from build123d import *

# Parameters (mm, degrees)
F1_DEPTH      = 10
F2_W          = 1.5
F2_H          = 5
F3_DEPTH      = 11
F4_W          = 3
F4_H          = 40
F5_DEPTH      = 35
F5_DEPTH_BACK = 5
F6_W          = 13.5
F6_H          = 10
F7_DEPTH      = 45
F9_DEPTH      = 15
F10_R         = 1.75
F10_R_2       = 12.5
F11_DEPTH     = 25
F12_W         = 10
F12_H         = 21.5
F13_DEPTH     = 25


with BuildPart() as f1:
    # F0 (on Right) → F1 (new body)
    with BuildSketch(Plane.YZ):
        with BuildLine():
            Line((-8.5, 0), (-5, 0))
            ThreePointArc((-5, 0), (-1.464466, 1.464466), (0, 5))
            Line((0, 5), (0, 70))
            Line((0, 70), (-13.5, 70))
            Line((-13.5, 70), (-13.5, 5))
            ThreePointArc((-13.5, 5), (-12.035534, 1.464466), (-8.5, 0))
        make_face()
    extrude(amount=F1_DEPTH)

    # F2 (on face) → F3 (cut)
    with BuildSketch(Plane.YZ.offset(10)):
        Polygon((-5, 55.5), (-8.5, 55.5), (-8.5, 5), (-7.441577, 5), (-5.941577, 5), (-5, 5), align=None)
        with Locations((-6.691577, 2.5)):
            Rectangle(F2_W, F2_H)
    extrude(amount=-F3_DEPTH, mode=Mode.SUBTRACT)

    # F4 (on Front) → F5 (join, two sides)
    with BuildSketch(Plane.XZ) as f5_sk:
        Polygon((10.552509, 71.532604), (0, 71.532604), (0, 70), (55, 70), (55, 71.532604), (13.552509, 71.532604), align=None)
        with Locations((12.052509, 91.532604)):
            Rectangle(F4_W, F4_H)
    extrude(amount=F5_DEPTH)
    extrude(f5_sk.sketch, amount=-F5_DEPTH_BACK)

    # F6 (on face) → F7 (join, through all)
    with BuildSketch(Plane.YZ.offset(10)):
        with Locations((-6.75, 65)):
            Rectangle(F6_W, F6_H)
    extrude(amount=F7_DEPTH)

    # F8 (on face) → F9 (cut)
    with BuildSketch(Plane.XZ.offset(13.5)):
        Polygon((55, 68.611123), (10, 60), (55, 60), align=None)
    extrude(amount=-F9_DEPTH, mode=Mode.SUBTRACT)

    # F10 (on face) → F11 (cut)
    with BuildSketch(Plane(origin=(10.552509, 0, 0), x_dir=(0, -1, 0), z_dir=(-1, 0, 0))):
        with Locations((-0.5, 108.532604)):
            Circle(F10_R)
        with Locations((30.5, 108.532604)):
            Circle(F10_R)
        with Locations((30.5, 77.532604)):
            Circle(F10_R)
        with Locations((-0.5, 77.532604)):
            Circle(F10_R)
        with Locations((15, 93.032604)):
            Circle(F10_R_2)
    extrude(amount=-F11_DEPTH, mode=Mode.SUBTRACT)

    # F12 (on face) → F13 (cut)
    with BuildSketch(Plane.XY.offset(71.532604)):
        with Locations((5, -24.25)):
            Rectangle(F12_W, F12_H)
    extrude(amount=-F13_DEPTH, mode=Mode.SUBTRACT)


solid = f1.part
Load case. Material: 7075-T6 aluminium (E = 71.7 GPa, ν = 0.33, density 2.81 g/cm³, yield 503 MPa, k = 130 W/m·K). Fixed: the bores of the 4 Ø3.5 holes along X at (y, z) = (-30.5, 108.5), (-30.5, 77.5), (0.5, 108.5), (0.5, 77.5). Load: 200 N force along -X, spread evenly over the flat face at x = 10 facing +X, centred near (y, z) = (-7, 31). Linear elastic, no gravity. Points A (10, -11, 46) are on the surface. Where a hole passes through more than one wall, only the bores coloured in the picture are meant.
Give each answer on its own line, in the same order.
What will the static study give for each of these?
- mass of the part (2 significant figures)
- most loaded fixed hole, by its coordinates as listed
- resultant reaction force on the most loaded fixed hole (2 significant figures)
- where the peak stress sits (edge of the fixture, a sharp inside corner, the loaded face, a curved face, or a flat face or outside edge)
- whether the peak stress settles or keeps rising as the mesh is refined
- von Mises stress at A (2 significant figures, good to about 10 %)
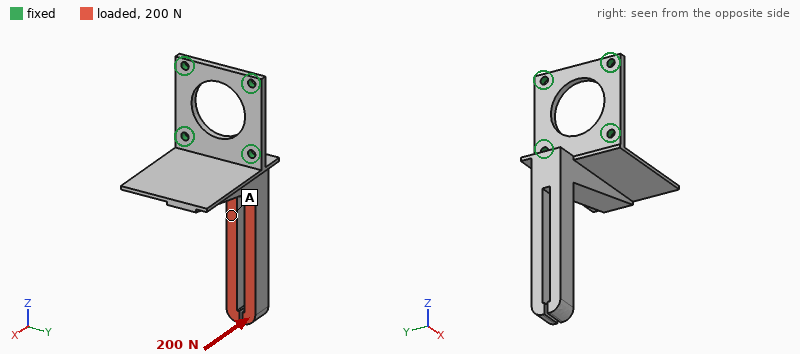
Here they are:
48 g
(0.5, 77.5)
140 N
edge of the fixture
keeps rising
21 MPa
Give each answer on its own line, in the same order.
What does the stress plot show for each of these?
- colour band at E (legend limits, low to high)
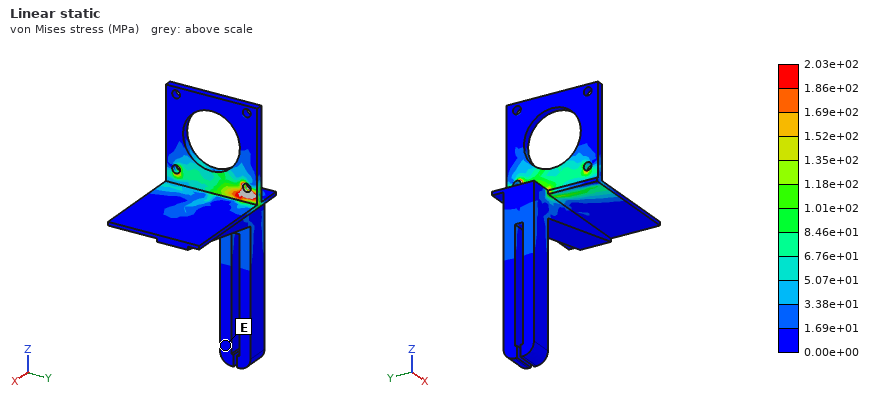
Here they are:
0.00e+00 to 1.69e+01 MPa
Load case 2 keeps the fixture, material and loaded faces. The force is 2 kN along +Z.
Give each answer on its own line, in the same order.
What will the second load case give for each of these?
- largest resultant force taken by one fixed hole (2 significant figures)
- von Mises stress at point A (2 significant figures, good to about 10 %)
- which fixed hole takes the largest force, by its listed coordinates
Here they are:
1.6 kN
60 MPa
(0.5, 77.5)
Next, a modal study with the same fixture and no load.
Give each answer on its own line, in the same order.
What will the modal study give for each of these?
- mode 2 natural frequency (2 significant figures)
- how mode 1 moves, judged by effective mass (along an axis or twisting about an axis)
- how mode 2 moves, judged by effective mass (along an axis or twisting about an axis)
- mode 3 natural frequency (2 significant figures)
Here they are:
1000 Hz
along X
along Y
1200 Hz
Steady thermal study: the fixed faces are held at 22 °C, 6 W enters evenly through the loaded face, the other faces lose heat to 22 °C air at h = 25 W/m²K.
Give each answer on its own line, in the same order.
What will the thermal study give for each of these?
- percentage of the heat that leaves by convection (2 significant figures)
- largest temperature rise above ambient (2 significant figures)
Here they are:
27 %
18 K
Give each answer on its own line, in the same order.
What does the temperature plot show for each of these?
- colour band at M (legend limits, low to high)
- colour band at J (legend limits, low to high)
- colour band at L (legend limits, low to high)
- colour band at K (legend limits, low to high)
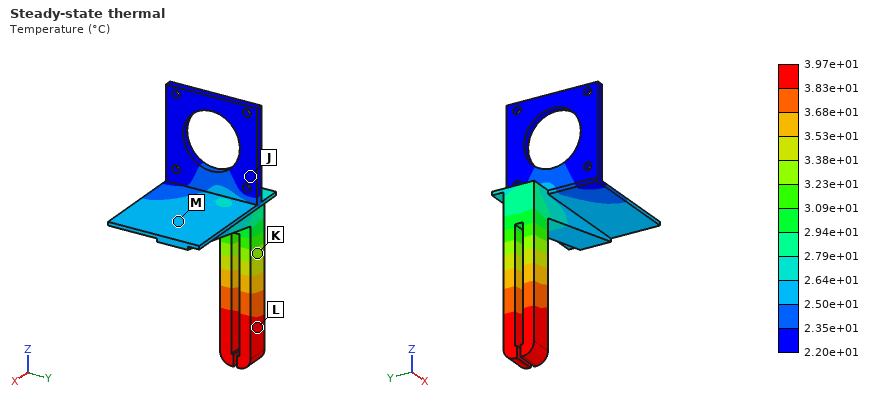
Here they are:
2.50e+01 to 2.64e+01 °C
2.20e+01 to 2.35e+01 °C
3.83e+01 to 3.97e+01 °C
3.23e+01 to 3.38e+01 °C
